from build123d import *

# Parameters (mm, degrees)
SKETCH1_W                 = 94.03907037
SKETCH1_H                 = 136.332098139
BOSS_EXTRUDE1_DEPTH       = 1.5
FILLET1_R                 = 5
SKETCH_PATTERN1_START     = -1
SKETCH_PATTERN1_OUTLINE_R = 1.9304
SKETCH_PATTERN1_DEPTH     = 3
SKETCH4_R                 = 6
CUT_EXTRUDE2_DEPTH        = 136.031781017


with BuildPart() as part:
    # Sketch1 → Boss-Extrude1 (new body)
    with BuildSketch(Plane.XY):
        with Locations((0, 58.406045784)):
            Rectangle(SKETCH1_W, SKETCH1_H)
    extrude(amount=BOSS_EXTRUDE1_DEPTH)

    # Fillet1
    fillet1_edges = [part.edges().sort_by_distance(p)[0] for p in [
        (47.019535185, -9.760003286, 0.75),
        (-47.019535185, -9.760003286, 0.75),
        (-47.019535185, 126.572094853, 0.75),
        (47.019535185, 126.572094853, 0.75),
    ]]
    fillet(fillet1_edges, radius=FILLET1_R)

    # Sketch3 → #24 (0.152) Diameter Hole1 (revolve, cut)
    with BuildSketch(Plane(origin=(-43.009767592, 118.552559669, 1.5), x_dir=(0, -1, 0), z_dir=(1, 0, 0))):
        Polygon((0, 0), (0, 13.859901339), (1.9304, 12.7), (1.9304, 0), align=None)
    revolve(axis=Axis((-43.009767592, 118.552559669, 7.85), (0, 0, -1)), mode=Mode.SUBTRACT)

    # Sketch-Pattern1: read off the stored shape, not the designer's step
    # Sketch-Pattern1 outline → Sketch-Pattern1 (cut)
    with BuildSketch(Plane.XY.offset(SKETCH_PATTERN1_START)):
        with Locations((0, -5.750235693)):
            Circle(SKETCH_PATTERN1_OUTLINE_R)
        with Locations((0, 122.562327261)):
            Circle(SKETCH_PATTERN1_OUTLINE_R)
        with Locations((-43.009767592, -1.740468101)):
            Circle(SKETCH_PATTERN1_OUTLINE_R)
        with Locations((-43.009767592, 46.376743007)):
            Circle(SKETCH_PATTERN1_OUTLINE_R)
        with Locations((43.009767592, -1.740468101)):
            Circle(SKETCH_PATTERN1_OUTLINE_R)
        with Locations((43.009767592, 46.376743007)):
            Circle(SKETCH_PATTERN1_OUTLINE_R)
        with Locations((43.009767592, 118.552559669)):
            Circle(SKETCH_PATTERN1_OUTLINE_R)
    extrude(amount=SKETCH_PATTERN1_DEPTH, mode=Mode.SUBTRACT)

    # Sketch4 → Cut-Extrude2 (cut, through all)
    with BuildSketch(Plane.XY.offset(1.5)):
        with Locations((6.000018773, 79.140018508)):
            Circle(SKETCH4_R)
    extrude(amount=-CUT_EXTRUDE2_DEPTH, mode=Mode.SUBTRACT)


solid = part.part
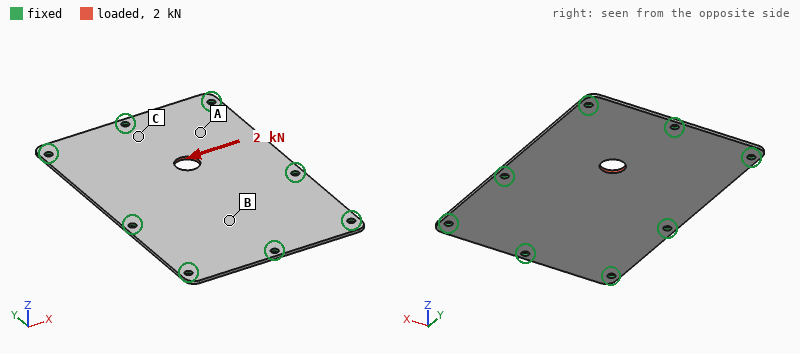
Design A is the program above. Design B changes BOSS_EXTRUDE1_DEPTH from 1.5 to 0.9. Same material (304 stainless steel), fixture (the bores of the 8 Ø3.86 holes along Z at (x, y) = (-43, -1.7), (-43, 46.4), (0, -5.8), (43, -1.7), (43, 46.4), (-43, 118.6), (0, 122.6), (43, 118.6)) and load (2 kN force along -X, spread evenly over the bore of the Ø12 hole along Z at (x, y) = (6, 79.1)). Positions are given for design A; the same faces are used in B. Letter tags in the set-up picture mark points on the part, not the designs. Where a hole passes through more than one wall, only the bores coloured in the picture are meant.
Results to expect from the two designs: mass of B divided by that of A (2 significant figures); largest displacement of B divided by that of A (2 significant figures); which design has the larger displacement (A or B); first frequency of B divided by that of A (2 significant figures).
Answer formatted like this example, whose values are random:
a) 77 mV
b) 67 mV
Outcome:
a) 0.60
b) 1.7
c) B
d) 0.61
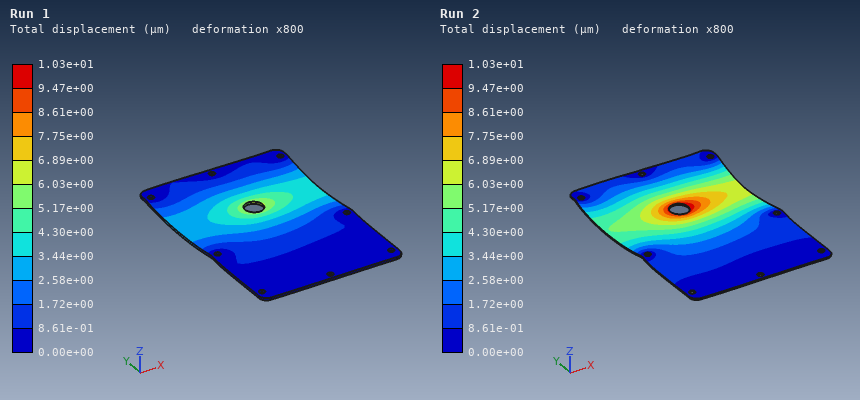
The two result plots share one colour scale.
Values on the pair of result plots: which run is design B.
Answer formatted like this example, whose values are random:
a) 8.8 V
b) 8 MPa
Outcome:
a) Run 2
